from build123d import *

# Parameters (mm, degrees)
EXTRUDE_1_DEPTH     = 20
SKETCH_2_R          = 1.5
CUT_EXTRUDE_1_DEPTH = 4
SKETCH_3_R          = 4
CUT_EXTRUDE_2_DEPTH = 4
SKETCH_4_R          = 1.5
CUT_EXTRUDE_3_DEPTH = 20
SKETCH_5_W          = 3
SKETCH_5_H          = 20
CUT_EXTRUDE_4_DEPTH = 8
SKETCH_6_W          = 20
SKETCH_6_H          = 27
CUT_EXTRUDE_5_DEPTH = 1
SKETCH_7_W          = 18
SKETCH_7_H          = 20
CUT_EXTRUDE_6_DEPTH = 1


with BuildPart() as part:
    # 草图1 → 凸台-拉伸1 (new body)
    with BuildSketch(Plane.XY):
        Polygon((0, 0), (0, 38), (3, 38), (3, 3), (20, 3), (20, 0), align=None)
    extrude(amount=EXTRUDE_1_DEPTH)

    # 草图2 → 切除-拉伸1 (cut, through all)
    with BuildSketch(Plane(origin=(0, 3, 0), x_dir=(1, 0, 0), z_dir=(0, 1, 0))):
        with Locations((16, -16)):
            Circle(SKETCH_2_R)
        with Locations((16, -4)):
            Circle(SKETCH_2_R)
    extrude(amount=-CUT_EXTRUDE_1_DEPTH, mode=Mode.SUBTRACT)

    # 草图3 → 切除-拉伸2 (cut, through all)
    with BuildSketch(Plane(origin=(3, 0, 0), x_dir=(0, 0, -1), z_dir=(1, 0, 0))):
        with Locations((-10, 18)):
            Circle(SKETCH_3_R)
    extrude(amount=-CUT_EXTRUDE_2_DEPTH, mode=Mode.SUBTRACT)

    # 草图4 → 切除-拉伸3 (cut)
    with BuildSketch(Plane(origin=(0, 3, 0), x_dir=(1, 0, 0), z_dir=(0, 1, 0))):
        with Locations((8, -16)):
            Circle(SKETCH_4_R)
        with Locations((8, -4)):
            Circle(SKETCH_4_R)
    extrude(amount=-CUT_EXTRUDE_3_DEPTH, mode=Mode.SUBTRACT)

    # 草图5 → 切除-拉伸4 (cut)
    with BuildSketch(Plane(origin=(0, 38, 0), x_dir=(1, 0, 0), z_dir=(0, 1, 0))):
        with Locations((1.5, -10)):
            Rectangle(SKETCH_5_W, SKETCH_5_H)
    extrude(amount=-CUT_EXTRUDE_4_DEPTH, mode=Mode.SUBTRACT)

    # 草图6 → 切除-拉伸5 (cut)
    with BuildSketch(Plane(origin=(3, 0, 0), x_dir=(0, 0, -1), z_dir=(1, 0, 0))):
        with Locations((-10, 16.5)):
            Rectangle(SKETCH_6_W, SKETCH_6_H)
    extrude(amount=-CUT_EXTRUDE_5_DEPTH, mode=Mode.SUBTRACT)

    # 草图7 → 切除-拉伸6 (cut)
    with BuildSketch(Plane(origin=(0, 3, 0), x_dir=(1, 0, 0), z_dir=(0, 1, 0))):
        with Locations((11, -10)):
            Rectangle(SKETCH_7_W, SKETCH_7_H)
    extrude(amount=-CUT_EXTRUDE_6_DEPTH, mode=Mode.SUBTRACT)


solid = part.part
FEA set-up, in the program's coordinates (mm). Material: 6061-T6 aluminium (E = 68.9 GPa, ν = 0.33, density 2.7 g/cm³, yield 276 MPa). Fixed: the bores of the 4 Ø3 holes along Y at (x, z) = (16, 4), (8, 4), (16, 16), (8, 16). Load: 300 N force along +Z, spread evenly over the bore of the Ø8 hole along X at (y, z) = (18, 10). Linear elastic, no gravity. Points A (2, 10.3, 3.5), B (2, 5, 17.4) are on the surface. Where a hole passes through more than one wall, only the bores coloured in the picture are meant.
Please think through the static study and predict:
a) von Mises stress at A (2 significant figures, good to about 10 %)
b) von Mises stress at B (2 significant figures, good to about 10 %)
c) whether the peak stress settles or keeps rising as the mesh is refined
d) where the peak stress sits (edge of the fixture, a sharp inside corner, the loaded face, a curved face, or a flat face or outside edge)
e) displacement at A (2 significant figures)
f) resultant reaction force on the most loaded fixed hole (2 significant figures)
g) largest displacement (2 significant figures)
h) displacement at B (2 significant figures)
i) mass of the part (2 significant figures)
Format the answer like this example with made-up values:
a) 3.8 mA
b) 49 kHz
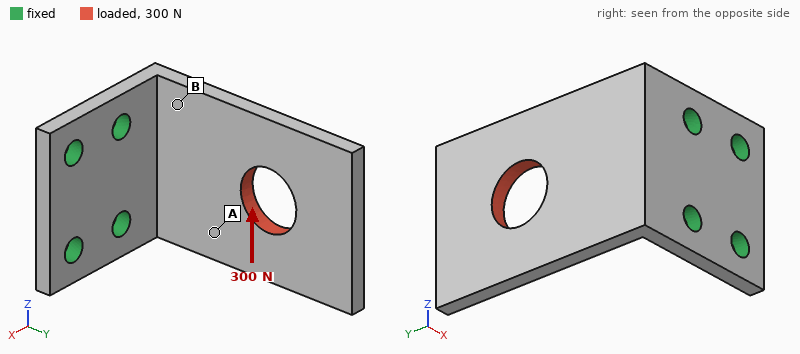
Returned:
a) 34 MPa
b) 87 MPa
c) keeps rising
d) edge of the fixture
e) 0.082 mm
f) 430 N
g) 0.22 mm
h) 0.055 mm
i) 4.8 g
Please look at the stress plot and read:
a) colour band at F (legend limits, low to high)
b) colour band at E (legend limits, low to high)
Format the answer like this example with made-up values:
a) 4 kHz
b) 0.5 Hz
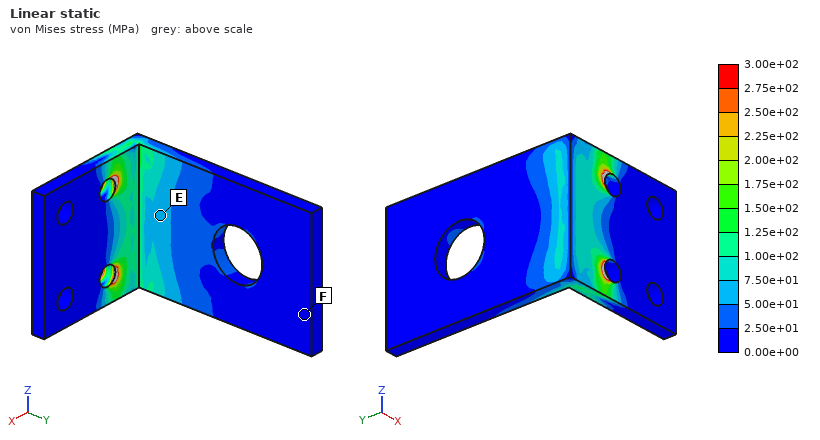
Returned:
a) 0.00e+00 to 2.50e+01 MPa
b) 5.00e+01 to 7.50e+01 MPa
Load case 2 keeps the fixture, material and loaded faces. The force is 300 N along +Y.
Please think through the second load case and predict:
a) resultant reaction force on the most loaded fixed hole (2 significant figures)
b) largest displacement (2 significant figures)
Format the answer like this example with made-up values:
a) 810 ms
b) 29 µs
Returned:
a) 170 N
b) 0.19 mm
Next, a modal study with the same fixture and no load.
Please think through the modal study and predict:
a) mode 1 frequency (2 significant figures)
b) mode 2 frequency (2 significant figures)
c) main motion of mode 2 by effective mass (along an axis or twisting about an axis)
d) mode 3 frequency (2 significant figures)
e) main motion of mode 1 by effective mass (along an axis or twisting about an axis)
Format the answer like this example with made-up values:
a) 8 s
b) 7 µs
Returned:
a) 1500 Hz
b) 4400 Hz
c) along Z
d) 6000 Hz
e) along X
